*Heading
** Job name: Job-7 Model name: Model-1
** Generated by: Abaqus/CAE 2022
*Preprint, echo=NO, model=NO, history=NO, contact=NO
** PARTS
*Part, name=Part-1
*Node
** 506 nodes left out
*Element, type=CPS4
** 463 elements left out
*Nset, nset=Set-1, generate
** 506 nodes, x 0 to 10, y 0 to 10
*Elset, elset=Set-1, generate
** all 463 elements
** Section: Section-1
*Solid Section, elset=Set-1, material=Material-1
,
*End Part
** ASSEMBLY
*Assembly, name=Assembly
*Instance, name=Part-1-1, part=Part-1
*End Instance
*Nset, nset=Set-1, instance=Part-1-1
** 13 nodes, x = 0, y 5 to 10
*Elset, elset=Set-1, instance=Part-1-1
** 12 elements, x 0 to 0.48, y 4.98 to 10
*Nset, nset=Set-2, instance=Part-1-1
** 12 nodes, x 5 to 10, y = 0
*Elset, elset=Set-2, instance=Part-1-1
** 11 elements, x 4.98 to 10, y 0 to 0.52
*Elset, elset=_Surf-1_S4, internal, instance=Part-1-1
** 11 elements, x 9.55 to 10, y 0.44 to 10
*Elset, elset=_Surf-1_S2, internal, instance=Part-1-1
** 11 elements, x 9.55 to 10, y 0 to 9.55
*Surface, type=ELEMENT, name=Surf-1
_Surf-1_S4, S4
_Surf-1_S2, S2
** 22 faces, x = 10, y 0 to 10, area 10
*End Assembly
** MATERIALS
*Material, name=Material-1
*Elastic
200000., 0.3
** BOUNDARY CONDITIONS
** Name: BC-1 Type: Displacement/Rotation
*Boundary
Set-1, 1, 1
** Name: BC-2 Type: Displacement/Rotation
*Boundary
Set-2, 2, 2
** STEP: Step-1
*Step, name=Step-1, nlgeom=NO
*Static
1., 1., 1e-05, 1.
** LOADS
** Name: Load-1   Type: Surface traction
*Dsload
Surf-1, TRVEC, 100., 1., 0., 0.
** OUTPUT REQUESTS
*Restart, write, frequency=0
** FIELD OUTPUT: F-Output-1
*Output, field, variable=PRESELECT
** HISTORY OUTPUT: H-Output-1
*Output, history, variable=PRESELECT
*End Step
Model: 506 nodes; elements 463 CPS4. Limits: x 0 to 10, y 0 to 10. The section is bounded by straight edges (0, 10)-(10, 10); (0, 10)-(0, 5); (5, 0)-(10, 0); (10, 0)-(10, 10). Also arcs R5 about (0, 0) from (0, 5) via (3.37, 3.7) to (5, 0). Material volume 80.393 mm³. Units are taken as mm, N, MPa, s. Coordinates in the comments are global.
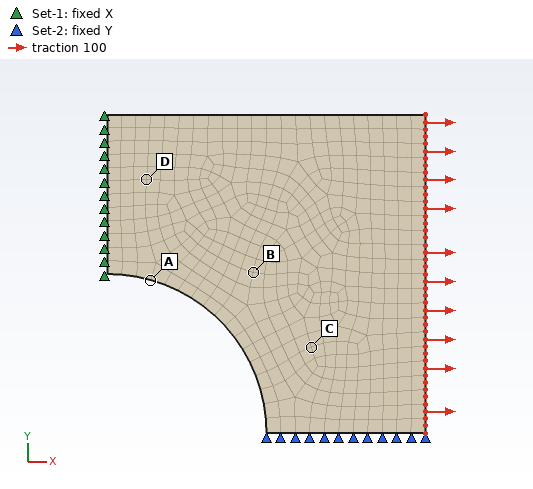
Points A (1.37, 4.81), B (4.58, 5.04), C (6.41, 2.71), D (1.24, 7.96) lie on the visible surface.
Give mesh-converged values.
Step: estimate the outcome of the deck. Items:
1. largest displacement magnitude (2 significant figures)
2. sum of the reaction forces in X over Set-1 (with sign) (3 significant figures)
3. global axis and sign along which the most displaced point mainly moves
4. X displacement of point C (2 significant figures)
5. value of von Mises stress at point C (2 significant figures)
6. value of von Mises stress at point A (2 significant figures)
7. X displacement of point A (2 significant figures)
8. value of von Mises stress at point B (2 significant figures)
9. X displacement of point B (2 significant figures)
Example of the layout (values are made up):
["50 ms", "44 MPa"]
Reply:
["0.019 mm", "-1000 N", "+X", "0.016 mm", "180 MPa", "540 MPa", "0.0044 mm", "230 MPa", "0.0084 mm"]
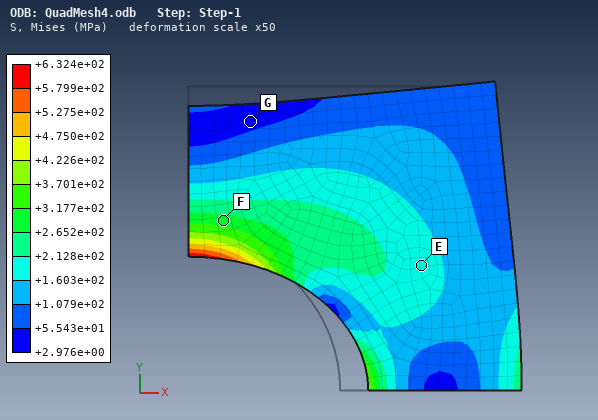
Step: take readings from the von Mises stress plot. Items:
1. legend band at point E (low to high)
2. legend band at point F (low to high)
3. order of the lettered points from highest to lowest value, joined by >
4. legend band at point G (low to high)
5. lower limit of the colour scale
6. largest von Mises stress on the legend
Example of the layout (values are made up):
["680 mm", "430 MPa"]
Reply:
["+1.603e+02 to +2.128e+02 MPa", "+2.652e+02 to +3.177e+02 MPa", "F > E > G", "+2.976e+00 to +5.543e+01 MPa", "+2.976e+00 MPa", "+6.324e+02 MPa"]
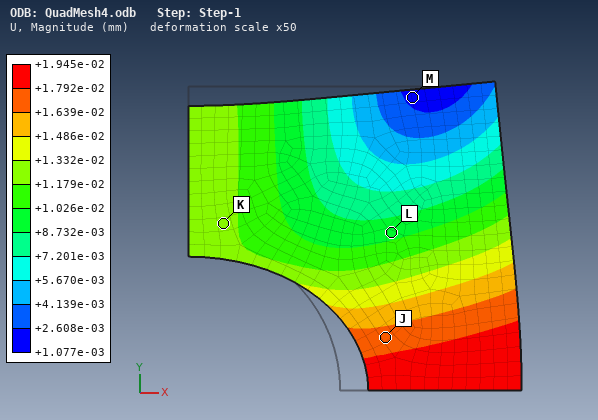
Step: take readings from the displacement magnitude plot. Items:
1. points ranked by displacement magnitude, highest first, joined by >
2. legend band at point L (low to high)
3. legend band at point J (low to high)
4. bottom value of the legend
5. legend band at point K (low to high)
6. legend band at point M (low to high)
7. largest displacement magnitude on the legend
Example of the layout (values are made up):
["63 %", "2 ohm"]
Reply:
["J > K > L > M", "+8.732e-03 to +1.026e-02 mm", "+1.639e-02 to +1.792e-02 mm", "+1.077e-03 mm", "+1.179e-02 to +1.332e-02 mm", "+1.077e-03 to +2.608e-03 mm", "+1.945e-02 mm"]
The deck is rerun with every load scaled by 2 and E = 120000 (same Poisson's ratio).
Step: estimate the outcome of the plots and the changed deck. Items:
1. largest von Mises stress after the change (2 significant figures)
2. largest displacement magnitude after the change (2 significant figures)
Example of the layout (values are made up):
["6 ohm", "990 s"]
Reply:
["1300 MPa", "0.065 mm"]
